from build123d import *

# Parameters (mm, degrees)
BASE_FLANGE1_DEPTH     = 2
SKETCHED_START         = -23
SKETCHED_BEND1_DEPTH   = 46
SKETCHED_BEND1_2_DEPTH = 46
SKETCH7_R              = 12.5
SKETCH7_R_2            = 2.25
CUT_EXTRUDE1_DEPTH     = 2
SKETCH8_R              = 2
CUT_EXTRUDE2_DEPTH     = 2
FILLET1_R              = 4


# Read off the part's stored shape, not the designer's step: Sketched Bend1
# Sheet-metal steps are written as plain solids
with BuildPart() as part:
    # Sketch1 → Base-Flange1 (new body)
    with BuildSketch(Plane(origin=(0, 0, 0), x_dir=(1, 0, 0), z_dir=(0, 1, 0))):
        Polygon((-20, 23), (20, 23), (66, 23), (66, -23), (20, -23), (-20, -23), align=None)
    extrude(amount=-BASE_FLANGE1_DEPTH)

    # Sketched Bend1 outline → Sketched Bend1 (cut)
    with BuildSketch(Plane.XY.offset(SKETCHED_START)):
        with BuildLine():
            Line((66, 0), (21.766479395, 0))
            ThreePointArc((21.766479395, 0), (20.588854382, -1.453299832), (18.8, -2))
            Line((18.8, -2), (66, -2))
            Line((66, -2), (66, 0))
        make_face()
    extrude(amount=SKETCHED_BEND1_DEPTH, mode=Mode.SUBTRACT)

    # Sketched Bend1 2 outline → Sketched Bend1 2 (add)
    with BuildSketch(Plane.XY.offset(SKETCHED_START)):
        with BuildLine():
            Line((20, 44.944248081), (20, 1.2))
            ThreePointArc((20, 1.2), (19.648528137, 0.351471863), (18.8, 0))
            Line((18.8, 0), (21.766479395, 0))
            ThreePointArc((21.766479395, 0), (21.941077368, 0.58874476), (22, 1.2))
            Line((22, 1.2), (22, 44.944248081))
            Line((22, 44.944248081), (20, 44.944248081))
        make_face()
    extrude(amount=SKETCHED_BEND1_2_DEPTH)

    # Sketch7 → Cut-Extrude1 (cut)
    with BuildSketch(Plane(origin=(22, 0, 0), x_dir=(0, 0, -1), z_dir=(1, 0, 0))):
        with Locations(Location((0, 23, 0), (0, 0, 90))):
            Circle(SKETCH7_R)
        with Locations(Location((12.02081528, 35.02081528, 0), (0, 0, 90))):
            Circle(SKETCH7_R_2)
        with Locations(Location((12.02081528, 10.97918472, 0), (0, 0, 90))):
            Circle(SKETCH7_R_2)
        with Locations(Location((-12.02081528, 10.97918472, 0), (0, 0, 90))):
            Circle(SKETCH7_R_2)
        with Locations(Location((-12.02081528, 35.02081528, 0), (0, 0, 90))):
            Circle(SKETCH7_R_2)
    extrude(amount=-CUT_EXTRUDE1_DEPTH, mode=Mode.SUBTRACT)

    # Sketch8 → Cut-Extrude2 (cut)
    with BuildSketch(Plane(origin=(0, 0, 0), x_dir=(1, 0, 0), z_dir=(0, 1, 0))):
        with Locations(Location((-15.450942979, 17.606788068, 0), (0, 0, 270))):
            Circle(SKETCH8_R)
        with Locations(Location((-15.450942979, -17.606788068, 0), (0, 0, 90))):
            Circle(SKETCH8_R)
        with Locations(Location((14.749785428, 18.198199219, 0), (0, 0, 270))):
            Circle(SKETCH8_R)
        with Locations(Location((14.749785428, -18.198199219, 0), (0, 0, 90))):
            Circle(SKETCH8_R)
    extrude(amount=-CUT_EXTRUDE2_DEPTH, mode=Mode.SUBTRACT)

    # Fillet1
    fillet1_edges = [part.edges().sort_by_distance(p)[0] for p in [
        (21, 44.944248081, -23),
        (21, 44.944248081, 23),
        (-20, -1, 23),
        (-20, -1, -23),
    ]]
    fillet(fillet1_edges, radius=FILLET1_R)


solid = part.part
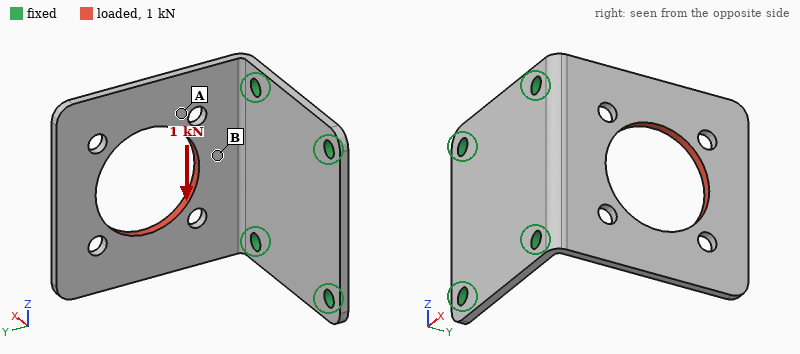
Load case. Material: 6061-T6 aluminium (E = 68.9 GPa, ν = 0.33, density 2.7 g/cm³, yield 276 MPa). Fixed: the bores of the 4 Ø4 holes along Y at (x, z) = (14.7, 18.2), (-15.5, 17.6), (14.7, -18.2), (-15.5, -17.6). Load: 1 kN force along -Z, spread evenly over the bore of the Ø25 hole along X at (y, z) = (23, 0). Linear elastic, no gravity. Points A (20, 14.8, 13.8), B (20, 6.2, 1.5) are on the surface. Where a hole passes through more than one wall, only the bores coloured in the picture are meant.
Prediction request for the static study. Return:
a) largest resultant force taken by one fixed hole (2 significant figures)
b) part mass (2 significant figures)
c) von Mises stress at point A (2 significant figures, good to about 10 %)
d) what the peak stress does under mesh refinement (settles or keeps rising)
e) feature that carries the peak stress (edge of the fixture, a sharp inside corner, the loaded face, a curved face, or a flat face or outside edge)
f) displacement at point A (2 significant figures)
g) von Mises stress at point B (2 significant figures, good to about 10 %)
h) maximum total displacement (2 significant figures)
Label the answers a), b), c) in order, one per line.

a) 820 N
b) 18 g
c) 41 MPa
d) keeps rising
e) edge of the fixture
f) 0.10 mm
g) 83 MPa
h) 0.26 mm
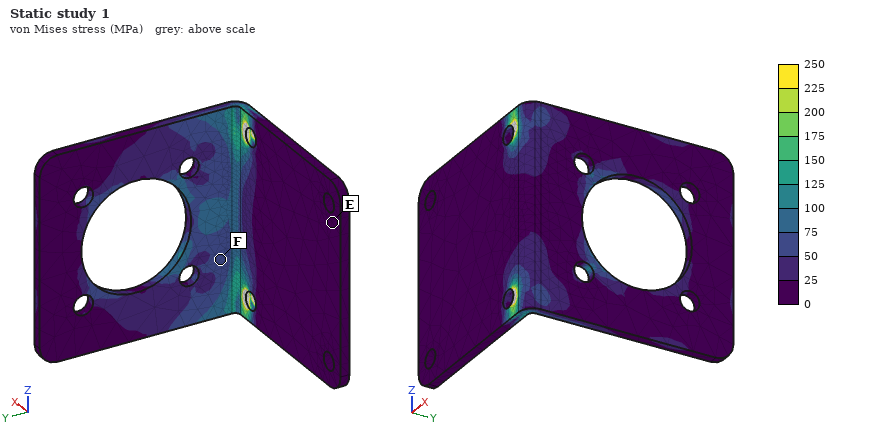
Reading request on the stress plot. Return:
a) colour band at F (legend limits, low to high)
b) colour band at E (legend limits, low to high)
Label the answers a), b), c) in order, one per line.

a) 50 to 75 MPa
b) 0 to 25 MPa
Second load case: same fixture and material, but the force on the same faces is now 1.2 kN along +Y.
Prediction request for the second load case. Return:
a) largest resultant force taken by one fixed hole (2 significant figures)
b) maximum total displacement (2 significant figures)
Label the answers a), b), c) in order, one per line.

a) 630 N
b) 0.47 mm
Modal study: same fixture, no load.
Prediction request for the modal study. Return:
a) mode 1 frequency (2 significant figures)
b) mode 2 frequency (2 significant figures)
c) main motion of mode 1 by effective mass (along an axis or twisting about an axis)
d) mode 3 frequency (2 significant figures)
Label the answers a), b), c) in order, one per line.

a) 630 Hz
b) 1500 Hz
c) along X
d) 3800 Hz
